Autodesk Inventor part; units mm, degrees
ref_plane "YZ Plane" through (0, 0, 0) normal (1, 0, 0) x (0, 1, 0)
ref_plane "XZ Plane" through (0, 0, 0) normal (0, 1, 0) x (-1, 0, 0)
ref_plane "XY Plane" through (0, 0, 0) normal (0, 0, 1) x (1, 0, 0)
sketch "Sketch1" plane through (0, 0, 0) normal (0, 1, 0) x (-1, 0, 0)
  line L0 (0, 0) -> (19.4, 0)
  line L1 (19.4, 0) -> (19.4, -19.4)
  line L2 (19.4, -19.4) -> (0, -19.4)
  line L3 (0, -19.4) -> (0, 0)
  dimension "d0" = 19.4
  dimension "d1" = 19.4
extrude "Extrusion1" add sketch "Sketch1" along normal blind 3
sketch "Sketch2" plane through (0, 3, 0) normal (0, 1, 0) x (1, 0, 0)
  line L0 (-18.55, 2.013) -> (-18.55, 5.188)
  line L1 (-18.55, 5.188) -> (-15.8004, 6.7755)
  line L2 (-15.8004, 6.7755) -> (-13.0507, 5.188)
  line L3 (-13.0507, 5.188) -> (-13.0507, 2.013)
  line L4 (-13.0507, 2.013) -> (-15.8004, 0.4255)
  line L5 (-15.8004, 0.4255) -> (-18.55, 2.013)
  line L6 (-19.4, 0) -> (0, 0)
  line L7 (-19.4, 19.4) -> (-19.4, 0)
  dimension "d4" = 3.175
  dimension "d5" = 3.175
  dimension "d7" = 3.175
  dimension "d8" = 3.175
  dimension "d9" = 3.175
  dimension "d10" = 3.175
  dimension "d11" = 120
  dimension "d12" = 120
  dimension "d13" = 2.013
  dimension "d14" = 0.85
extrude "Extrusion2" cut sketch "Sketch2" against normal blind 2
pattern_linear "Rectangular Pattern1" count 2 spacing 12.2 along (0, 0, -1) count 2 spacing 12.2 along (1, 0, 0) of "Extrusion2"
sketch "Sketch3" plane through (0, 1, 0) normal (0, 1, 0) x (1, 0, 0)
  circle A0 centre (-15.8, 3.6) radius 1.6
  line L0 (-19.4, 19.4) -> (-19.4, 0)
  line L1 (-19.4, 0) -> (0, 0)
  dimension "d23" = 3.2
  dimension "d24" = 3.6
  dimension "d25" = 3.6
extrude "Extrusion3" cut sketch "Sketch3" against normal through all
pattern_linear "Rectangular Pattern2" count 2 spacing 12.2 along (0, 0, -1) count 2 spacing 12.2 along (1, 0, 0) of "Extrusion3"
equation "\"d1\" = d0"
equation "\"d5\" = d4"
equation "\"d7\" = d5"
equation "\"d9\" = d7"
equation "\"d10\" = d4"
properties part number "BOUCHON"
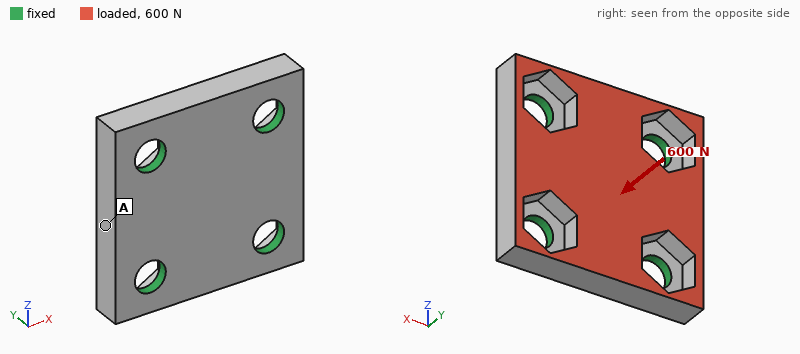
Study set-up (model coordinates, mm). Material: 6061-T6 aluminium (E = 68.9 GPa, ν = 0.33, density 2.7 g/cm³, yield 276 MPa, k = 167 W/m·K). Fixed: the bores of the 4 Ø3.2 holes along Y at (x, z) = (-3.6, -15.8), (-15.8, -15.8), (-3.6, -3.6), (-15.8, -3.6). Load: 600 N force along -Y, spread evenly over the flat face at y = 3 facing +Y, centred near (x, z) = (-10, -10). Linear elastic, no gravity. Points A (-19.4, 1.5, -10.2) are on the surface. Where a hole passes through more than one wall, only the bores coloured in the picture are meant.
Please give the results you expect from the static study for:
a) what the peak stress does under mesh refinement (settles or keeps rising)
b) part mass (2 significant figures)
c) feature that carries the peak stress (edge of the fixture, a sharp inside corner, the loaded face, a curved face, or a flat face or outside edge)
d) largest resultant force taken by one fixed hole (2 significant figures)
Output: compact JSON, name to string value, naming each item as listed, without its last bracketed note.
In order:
{"what the peak stress does under mesh refinement": "keeps rising", "part mass": "2.4 g", "feature that carries the peak stress": "edge of the fixture", "largest resultant force taken by one fixed hole": "160 N"}
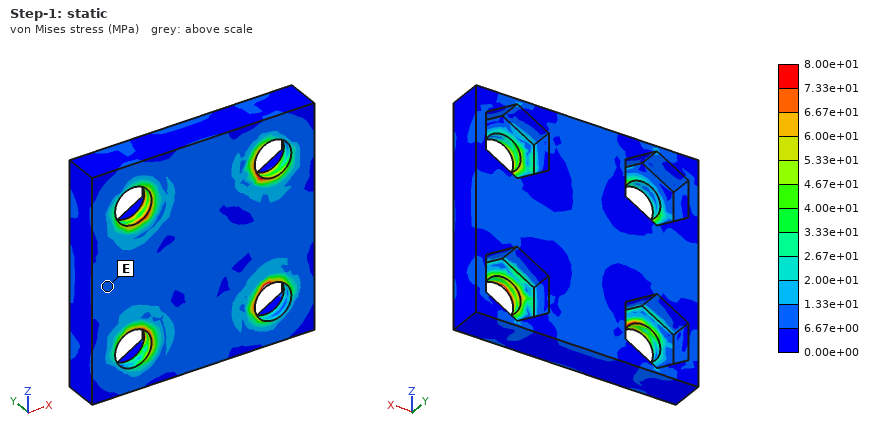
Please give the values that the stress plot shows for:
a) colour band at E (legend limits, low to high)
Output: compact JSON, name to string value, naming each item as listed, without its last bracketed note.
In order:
{"colour band at E": "6.67e+00 to 1.33e+01 MPa"}
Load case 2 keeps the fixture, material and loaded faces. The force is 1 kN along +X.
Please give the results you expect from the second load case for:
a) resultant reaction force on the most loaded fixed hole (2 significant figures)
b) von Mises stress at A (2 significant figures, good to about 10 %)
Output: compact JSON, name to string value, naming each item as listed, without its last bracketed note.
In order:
{"resultant reaction force on the most loaded fixed hole": "270 N", "von Mises stress at A": "5.9 MPa"}
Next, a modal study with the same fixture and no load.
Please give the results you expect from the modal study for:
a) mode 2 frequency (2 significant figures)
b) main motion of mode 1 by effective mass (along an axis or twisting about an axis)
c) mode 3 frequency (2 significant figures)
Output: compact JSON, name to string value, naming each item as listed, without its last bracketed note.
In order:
{"mode 2 frequency": "59 kHz", "main motion of mode 1 by effective mass": "along Y", "mode 3 frequency": "59 kHz"}
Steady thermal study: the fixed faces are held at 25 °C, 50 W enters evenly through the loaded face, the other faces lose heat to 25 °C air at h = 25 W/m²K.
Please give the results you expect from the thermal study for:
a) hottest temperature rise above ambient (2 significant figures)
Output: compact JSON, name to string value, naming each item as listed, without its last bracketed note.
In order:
{"hottest temperature rise above ambient": "17 K"}
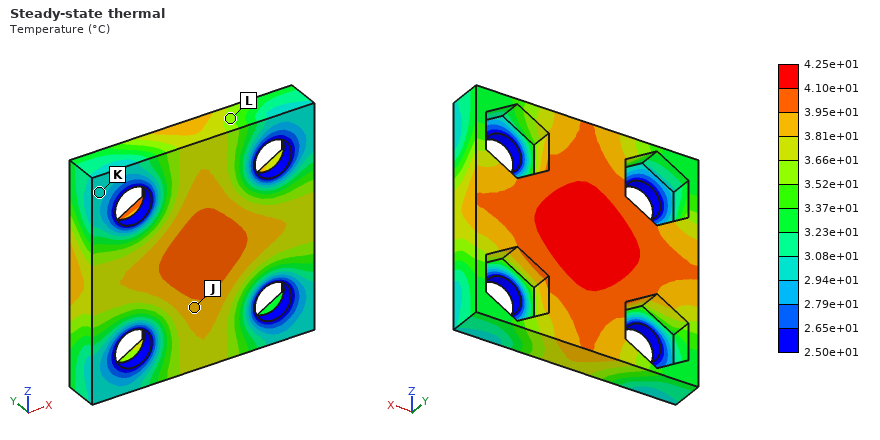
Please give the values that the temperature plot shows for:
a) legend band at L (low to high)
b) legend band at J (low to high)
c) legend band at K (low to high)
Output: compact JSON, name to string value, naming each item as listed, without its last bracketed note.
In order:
{"legend band at L": "3.52e+01 to 3.66e+01 °C", "legend band at J": "3.81e+01 to 3.95e+01 °C", "legend band at K": "2.94e+01 to 3.08e+01 °C"}
